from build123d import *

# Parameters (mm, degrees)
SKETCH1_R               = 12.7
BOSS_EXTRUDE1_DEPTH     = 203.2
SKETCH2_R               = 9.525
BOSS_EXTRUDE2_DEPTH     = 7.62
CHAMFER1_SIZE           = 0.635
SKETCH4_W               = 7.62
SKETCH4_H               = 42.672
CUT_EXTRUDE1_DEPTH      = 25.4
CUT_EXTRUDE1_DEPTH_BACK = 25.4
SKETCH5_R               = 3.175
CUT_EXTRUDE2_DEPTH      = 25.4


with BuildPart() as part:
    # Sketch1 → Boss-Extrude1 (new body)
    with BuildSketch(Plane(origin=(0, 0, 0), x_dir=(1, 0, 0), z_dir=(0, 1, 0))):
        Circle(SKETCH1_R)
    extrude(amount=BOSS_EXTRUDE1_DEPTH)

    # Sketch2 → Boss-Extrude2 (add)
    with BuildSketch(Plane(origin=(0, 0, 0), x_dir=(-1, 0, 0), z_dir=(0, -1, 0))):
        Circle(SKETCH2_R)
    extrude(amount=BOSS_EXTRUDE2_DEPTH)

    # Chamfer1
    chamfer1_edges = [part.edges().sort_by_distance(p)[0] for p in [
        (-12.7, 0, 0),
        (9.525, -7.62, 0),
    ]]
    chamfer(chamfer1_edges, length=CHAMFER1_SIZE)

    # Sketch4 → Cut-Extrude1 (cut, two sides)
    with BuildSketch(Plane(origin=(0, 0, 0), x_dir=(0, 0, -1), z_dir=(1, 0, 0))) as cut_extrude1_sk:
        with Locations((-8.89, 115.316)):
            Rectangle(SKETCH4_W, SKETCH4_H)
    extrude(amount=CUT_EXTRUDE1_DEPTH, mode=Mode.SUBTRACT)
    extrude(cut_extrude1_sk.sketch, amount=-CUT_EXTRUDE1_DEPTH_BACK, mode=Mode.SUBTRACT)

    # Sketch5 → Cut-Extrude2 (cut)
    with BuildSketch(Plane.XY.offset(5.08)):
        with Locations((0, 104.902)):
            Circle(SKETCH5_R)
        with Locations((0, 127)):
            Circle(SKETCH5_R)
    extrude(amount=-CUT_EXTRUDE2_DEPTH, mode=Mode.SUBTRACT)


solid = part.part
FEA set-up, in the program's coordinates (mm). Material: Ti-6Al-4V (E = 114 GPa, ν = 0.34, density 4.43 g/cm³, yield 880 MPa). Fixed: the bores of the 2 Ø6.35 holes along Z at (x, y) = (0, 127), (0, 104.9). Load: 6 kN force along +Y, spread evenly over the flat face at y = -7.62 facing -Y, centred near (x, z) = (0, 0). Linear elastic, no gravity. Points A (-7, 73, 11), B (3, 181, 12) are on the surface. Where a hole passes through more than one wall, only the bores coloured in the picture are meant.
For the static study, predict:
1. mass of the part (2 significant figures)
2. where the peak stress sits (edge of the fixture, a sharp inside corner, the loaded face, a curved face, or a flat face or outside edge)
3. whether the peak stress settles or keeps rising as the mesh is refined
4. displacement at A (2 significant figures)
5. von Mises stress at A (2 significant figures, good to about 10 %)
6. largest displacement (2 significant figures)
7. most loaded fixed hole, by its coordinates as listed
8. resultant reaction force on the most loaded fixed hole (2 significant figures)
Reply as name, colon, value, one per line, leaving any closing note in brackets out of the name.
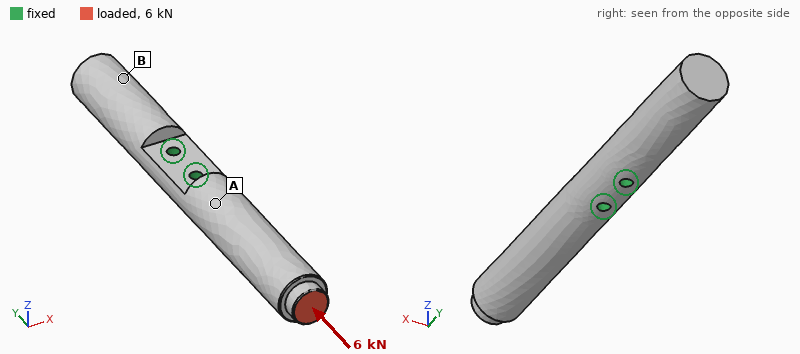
mass of the part: 440 g
where the peak stress sits: edge of the fixture
whether the peak stress settles or keeps rising as the mesh is refined: keeps rising
displacement at A: 11 µm
von Mises stress at A: 12 MPa
largest displacement: 35 µm
most loaded fixed hole, by its coordinates as listed: (0, 104.9)
resultant reaction force on the most loaded fixed hole: 5.2 kN
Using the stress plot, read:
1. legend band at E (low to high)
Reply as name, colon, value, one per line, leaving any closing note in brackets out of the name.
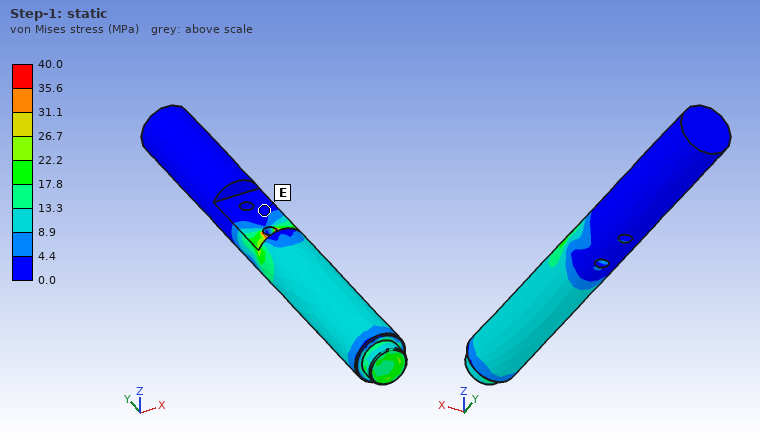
legend band at E: 0.0 to 4.4 MPa
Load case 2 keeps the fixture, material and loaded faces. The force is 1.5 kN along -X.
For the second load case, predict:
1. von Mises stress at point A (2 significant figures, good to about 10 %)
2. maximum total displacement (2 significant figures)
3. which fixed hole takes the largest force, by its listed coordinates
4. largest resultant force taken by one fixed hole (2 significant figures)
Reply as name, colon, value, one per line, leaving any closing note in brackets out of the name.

von Mises stress at point A: 39 MPa
maximum total displacement: 0.42 mm
which fixed hole takes the largest force, by its listed coordinates: (0, 104.9)
largest resultant force taken by one fixed hole: 5.7 kN
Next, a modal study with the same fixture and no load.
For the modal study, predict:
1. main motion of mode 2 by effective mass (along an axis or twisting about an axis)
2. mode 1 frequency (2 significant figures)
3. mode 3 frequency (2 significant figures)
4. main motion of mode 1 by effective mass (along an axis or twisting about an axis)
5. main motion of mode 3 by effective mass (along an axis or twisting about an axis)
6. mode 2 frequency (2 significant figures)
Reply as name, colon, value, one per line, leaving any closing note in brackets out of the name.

main motion of mode 2 by effective mass: along X
mode 1 frequency: 1100 Hz
mode 3 frequency: 2200 Hz
main motion of mode 1 by effective mass: along Z
main motion of mode 3 by effective mass: along Z
mode 2 frequency: 1200 Hz
